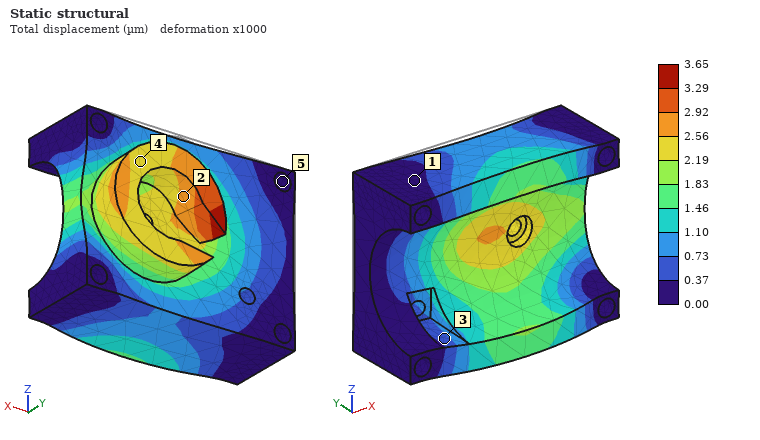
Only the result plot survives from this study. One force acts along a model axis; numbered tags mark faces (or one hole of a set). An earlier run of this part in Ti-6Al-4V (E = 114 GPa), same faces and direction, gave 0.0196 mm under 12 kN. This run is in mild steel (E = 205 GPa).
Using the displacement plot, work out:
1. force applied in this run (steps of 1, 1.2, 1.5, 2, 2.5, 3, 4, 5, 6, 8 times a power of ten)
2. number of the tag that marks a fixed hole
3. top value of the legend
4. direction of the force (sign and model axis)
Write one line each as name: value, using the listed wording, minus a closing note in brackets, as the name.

force applied in this run: 4 kN
number of the tag that marks a fixed hole: 5
top value of the legend: 3.65 µm
direction of the force: -Y
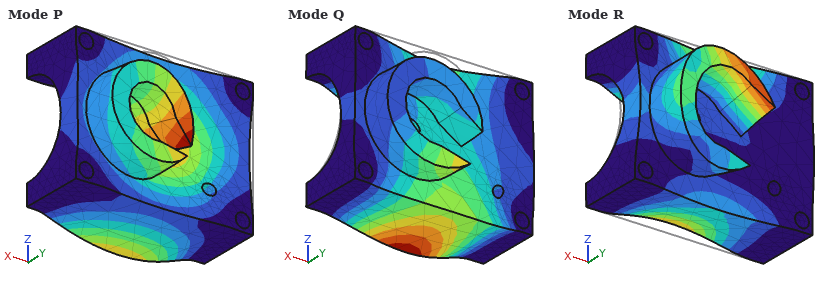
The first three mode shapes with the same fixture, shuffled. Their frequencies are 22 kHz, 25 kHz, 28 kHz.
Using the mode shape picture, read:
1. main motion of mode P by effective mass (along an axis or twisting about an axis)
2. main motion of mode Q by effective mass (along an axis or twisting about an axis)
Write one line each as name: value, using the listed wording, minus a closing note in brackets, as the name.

main motion of mode P by effective mass: along Y
main motion of mode Q by effective mass: along Z
